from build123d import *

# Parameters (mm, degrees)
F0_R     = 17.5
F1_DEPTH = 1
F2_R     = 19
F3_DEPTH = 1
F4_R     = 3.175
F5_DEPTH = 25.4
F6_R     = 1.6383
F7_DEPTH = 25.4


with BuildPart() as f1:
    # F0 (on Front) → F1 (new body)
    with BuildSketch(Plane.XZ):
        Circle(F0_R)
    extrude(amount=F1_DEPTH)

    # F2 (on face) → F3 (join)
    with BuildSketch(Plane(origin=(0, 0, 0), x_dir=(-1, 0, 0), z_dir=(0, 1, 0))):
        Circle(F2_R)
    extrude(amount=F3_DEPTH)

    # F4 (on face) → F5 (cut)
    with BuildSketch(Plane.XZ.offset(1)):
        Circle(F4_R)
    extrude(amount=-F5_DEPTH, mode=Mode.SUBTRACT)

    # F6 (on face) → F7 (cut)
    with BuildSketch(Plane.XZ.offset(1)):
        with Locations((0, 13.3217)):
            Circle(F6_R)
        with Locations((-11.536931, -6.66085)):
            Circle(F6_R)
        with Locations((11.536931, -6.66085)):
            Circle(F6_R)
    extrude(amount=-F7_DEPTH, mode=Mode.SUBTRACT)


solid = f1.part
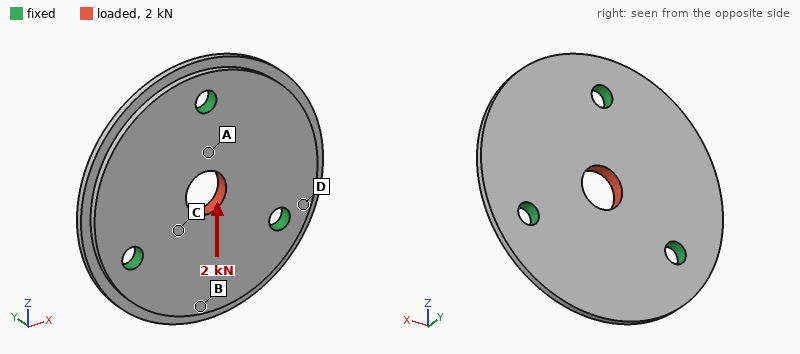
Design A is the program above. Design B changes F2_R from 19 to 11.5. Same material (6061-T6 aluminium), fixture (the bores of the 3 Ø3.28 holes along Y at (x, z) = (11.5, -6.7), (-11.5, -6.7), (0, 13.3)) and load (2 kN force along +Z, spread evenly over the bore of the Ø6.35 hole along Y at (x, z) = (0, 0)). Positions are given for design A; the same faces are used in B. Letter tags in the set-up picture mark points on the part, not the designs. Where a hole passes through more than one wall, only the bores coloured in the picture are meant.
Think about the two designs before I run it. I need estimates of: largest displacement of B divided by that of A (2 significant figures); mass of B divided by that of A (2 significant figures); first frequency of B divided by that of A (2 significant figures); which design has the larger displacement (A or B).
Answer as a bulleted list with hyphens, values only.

- 3.7
- 0.65
- 1.5
- B
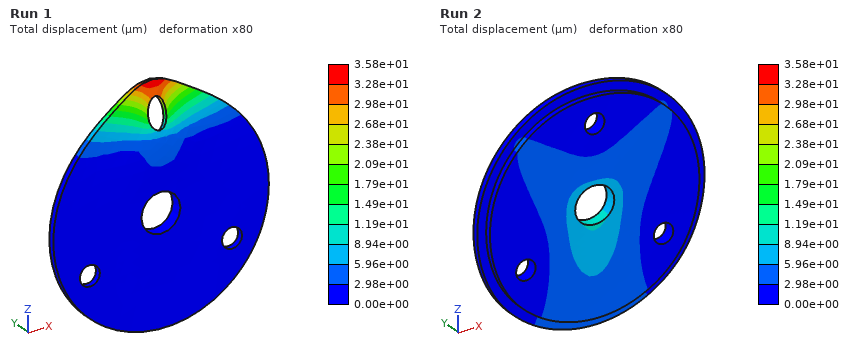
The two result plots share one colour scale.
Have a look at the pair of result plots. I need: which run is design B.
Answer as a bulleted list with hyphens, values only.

- Run 1
